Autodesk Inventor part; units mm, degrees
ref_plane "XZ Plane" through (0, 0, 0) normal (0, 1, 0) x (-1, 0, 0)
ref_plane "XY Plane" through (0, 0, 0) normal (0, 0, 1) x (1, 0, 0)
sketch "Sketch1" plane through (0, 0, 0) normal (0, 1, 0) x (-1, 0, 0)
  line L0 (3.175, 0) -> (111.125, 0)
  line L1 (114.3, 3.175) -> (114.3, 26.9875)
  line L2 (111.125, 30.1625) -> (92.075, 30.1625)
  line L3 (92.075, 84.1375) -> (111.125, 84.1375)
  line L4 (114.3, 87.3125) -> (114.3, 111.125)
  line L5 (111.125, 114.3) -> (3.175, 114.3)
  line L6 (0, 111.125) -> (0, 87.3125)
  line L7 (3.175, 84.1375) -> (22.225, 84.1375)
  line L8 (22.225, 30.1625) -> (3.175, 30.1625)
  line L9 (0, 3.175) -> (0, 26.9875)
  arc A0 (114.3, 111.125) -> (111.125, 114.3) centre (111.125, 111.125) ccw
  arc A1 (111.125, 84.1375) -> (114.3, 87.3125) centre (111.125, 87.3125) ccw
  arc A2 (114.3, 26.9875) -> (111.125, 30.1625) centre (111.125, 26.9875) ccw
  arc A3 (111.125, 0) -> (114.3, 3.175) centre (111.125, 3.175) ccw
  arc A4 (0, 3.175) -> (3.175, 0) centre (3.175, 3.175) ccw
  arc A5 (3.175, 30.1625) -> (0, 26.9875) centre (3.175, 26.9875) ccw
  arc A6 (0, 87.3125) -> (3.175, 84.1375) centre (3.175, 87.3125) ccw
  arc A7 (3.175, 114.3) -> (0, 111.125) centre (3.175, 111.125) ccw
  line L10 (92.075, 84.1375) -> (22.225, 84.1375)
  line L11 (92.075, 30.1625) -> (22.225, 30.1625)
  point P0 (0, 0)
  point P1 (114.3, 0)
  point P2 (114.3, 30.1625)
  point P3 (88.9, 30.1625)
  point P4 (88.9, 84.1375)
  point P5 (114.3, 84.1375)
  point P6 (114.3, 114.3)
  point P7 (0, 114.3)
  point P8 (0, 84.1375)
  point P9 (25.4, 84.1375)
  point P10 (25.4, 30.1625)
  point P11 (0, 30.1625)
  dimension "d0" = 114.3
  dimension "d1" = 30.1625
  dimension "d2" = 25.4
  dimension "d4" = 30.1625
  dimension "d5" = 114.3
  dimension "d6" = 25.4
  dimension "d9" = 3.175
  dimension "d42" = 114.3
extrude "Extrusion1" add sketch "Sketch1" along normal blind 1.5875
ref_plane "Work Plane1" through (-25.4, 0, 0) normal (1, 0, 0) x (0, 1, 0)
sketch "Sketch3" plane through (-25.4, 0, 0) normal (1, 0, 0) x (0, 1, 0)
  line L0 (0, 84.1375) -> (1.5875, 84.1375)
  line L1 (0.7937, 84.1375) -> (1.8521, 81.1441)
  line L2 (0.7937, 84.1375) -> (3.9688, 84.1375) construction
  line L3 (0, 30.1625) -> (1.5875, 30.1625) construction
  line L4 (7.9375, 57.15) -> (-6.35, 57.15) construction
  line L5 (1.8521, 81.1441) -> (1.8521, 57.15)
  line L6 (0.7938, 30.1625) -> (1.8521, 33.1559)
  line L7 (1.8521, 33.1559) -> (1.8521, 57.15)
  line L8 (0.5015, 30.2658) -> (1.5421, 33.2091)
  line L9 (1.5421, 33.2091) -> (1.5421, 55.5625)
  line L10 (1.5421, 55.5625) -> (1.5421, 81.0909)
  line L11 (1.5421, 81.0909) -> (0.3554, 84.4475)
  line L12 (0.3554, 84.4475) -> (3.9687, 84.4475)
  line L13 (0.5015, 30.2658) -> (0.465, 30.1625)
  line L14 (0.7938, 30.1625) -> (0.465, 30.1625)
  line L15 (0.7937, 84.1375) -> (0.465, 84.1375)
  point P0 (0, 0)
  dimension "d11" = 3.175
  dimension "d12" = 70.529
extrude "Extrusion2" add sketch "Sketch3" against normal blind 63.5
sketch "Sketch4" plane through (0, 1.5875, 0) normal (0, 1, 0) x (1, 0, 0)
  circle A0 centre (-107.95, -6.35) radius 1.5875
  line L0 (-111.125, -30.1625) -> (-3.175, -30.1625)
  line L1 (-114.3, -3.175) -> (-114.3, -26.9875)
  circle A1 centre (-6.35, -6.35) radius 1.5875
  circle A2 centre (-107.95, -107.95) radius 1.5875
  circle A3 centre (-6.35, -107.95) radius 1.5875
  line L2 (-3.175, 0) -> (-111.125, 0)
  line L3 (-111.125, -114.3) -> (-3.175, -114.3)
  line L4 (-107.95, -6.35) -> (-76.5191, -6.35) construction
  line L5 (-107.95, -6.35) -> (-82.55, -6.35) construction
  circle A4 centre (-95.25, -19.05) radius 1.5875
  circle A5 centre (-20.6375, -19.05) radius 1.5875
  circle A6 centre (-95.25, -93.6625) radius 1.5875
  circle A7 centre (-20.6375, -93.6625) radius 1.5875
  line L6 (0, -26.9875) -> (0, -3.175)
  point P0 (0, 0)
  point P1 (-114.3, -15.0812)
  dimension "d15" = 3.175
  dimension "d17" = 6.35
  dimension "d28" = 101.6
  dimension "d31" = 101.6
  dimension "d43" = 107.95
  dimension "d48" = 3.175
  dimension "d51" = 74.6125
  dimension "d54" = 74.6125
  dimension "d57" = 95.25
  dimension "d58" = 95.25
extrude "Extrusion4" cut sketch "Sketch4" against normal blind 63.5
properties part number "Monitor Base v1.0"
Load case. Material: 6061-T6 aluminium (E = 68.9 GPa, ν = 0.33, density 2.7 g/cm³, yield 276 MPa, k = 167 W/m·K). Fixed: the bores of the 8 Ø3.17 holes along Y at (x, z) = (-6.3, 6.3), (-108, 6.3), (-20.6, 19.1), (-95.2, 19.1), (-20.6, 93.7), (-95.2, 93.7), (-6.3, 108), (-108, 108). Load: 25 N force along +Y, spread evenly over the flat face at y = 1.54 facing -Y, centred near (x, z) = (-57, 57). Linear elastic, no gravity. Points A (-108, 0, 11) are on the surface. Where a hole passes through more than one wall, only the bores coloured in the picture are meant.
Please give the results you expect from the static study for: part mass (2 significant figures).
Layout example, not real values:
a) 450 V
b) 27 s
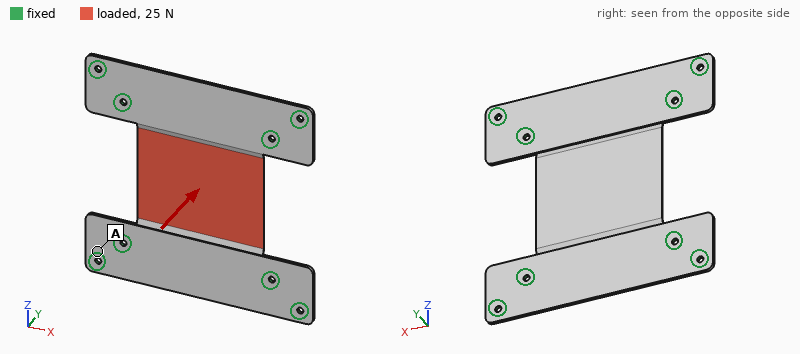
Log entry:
a) 32 g
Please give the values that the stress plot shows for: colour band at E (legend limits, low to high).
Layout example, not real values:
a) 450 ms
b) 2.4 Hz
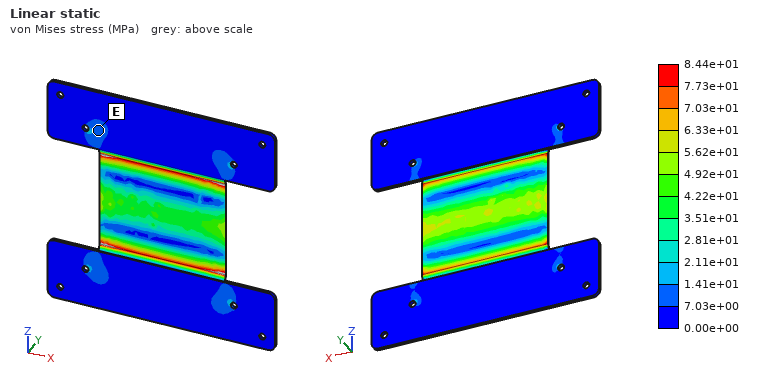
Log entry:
a) 7.03e+00 to 1.41e+01 MPa
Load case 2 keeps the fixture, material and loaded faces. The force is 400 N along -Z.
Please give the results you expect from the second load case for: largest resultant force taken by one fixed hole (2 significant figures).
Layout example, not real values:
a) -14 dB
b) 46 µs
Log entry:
a) 120 N
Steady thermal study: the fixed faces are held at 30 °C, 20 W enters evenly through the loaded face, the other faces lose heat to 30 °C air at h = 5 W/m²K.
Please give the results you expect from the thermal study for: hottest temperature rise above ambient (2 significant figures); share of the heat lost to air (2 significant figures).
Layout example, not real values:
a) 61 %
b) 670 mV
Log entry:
a) 61 K
b) 6.8 %
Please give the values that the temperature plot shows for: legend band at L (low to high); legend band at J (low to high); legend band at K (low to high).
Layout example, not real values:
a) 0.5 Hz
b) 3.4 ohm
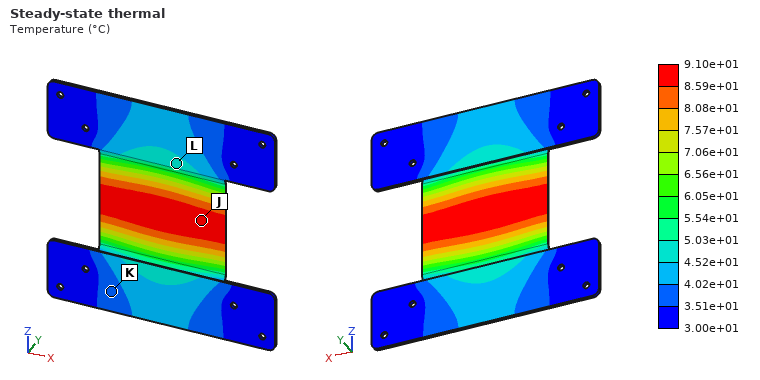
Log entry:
a) 4.52e+01 to 5.03e+01 °C
b) 8.59e+01 to 9.10e+01 °C
c) 3.51e+01 to 4.02e+01 °C
